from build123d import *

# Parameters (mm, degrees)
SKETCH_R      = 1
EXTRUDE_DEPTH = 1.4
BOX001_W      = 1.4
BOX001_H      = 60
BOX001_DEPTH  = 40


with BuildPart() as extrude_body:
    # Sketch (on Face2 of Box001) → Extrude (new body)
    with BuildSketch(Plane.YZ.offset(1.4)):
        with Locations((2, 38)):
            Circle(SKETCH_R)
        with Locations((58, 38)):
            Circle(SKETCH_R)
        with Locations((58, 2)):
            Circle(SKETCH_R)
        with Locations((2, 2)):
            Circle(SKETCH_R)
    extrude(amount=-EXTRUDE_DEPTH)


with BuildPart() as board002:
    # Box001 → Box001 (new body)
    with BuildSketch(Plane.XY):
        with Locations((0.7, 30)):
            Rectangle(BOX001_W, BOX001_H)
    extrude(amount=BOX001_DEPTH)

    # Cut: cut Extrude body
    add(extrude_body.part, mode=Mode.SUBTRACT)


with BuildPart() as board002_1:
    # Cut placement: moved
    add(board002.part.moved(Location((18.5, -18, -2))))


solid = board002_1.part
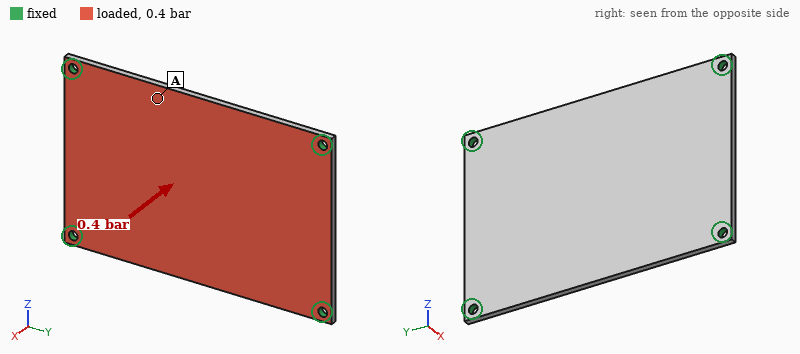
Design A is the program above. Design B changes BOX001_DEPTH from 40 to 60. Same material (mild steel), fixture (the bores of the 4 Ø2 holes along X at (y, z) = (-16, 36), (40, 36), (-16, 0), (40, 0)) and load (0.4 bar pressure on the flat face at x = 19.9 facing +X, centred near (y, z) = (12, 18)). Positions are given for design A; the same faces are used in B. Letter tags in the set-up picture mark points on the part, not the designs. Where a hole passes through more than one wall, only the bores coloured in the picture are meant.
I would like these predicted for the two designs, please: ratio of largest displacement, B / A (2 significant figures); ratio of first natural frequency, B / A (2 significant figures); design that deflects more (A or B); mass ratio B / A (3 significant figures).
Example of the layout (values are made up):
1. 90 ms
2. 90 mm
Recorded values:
1. 2.1
2. 0.77
3. B
4. 1.50
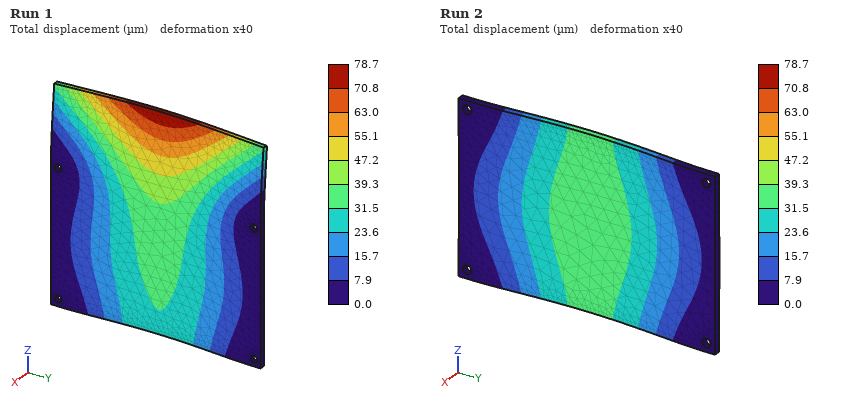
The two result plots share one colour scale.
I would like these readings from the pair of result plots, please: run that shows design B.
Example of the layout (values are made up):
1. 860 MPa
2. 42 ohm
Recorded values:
1. Run 1
